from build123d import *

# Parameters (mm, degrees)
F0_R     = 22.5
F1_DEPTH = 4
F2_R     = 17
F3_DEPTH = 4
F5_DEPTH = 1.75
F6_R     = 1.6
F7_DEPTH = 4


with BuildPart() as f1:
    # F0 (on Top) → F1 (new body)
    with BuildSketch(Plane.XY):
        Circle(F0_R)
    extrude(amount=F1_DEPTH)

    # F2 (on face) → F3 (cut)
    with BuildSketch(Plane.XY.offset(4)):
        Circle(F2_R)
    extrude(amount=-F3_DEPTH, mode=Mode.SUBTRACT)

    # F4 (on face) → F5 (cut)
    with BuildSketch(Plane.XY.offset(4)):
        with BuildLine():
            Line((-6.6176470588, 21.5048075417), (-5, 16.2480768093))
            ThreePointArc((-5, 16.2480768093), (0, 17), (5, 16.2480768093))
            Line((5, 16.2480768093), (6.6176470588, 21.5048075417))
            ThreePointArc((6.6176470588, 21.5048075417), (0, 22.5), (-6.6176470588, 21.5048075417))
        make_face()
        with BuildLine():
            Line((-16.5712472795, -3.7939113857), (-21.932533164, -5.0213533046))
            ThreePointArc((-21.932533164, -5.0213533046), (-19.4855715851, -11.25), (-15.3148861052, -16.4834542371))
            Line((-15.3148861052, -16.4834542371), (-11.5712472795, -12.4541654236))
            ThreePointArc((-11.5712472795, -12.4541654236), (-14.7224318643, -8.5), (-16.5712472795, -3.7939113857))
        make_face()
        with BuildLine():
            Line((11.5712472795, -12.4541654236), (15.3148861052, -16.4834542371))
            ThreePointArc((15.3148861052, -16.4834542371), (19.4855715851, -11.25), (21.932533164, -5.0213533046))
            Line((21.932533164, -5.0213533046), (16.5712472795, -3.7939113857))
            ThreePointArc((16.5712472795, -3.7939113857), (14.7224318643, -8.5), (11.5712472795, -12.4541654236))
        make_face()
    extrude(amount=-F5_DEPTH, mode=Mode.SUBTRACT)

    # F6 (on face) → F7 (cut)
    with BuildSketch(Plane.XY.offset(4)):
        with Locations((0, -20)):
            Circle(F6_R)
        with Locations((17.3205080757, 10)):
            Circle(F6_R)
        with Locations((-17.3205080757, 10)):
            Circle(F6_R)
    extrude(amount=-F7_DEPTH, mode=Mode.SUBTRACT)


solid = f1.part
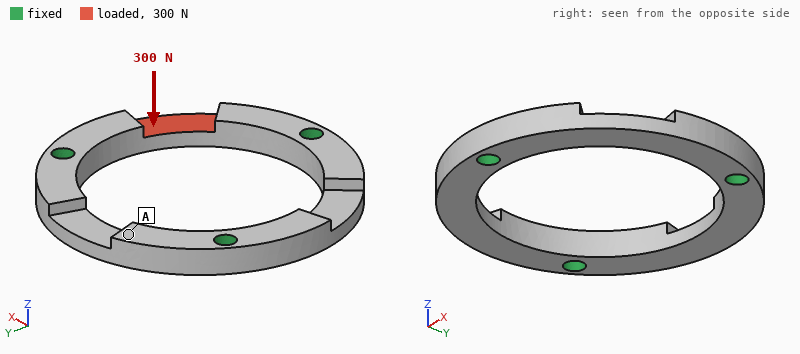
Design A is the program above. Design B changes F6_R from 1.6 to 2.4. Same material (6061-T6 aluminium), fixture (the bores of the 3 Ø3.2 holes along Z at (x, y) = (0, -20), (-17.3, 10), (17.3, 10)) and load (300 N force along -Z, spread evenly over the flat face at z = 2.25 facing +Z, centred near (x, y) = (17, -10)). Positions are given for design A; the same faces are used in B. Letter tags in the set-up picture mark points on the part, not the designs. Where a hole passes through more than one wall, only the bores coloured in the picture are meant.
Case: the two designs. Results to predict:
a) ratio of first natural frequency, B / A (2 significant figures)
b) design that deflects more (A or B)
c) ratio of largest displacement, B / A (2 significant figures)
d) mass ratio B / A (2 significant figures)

1.1
A
0.86
0.95
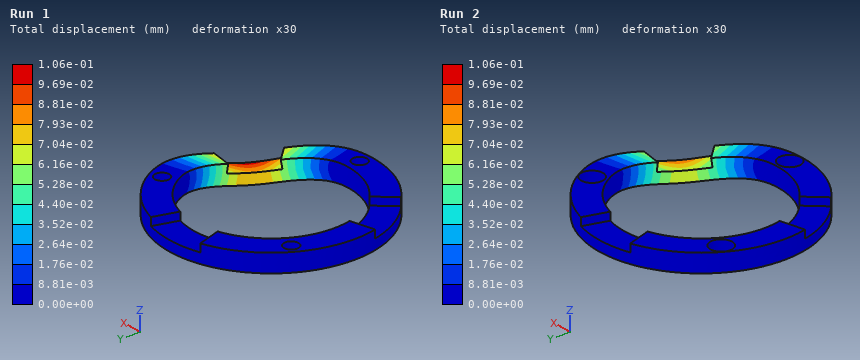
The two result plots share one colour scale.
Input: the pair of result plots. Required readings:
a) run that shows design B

Run 2
